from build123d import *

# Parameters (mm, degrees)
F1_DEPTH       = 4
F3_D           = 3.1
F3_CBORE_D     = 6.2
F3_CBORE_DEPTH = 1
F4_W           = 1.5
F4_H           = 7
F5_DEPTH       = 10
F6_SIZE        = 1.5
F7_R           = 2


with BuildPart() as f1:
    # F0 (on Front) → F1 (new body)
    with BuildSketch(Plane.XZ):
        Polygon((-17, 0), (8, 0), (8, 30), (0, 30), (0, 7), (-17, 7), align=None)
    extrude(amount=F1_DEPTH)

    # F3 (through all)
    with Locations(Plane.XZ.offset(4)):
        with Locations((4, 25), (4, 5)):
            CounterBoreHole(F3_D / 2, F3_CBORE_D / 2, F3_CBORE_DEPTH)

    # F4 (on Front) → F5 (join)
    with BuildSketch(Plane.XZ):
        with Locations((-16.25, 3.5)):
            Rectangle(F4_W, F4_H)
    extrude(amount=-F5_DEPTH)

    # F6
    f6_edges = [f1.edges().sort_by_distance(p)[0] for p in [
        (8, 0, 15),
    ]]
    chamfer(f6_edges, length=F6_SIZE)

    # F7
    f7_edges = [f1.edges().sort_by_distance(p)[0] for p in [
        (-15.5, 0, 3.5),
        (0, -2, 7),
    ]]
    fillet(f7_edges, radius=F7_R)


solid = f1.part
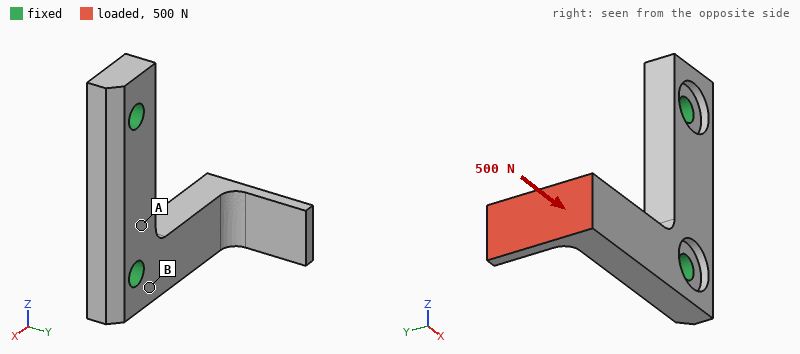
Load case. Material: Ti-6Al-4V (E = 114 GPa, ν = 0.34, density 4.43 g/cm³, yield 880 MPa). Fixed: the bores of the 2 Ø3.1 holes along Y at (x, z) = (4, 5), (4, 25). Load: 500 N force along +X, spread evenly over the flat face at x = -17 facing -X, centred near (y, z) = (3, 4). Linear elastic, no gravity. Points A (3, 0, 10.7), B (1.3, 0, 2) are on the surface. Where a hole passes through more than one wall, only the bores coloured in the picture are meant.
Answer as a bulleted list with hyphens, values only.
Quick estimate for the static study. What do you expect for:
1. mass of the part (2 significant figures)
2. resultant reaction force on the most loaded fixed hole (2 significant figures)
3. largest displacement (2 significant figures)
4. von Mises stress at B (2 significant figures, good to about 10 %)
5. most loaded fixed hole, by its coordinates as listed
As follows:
- 6.3 g
- 520 N
- 0.35 mm
- 130 MPa
- (4, 5)
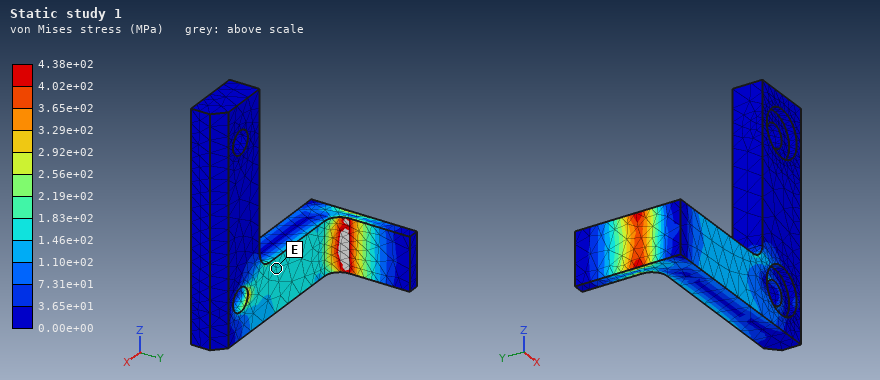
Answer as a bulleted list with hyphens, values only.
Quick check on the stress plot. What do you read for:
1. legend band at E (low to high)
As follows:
- 1.46e+02 to 1.83e+02 MPa
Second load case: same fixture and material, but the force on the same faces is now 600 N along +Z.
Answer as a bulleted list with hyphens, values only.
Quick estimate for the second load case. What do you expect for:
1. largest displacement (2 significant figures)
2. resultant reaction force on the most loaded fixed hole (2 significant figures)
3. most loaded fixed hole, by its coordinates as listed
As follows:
- 0.35 mm
- 470 N
- (4, 5)
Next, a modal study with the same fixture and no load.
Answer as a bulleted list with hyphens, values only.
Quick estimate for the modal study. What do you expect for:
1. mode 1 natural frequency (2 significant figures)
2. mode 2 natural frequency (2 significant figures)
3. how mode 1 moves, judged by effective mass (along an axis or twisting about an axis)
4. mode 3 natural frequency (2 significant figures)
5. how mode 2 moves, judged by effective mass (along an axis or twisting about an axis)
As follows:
- 5200 Hz
- 8500 Hz
- along Y
- 12 kHz
- along Z
